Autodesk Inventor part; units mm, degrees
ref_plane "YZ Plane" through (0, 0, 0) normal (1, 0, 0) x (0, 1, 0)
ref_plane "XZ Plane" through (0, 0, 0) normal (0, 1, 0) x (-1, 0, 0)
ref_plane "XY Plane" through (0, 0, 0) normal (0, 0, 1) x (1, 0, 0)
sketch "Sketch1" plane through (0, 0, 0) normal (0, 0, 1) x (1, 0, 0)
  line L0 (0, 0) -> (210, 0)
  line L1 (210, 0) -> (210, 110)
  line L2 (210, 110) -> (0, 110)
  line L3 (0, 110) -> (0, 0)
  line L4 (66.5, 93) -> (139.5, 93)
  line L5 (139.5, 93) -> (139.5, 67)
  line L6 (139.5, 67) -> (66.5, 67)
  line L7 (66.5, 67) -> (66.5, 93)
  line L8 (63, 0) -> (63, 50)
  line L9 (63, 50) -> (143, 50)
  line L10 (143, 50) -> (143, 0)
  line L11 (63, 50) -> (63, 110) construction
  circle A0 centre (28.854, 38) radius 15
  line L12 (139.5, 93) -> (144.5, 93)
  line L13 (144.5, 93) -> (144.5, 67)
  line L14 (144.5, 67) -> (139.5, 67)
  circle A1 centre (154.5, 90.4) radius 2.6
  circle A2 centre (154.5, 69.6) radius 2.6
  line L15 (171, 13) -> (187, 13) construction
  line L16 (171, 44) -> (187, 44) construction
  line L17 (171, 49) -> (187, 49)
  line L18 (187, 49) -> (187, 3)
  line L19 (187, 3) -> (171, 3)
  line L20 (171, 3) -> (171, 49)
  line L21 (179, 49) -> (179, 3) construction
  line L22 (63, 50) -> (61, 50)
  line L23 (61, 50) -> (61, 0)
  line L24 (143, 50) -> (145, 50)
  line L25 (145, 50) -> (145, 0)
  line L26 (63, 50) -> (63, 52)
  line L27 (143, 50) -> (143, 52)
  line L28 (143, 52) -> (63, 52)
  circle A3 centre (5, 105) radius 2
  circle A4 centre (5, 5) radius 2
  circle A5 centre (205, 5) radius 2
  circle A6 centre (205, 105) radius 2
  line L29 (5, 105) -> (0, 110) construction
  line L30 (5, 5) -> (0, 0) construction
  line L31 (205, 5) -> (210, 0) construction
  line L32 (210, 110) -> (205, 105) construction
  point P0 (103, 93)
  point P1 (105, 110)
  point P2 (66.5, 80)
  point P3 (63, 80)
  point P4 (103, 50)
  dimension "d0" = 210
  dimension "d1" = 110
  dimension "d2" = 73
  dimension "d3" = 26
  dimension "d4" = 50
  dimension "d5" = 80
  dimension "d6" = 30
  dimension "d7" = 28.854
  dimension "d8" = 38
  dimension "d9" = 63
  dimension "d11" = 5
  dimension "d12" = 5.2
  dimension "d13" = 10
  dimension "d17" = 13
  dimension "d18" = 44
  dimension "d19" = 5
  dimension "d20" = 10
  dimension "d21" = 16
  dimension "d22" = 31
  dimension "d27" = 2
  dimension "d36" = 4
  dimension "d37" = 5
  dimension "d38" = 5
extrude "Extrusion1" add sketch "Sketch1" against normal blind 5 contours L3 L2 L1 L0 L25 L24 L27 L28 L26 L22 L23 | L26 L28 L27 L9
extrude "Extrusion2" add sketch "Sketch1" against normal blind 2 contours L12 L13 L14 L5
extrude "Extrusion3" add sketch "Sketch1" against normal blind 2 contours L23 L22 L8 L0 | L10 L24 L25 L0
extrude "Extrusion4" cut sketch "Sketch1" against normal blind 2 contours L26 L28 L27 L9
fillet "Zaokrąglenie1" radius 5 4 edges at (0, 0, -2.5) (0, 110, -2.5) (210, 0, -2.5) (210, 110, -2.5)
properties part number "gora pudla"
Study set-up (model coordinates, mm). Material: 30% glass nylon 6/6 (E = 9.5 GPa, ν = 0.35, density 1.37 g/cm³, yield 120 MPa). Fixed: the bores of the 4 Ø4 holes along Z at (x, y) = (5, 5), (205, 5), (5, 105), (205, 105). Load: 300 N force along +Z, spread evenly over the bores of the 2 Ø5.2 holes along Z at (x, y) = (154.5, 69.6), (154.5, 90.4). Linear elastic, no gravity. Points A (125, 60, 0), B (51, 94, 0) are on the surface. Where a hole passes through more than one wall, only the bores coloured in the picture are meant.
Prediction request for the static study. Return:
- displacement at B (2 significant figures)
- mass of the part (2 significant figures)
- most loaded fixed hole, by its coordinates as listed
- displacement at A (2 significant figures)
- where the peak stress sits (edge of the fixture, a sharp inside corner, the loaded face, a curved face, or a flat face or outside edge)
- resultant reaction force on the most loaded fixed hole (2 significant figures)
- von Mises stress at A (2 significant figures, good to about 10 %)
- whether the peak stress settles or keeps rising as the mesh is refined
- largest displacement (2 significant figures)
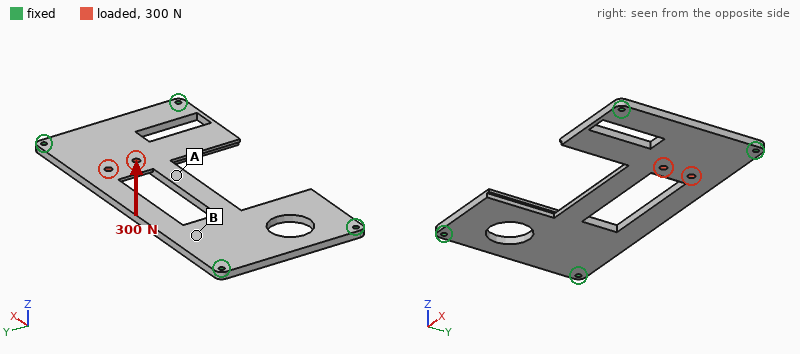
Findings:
0.75 mm
110 g
(205, 105)
2.1 mm
edge of the fixture
190 N
23 MPa
keeps rising
2.2 mm
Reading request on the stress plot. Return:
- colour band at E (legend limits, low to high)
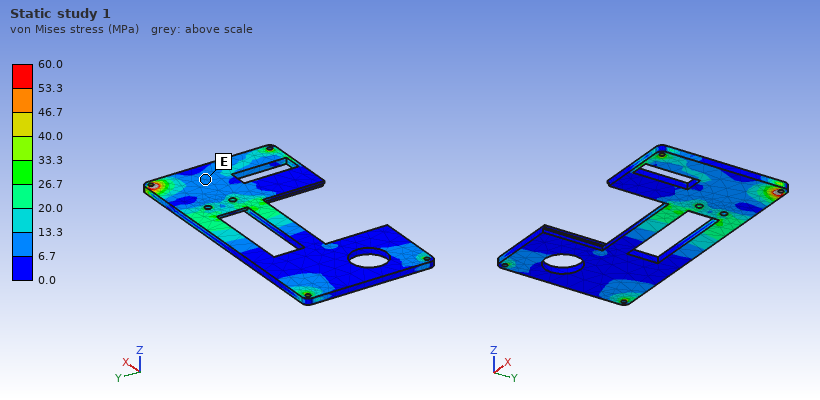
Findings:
6.7 to 13.3 MPa
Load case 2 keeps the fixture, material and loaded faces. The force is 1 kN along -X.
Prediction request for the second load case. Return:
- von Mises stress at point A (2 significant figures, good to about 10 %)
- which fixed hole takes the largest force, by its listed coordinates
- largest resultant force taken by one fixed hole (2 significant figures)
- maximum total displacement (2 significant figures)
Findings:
2.6 MPa
(205, 105)
580 N
49 µm
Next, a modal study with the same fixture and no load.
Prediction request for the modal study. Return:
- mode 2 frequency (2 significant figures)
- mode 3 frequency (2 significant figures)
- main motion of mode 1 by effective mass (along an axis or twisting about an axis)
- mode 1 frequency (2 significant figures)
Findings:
580 Hz
630 Hz
along Z
290 Hz
